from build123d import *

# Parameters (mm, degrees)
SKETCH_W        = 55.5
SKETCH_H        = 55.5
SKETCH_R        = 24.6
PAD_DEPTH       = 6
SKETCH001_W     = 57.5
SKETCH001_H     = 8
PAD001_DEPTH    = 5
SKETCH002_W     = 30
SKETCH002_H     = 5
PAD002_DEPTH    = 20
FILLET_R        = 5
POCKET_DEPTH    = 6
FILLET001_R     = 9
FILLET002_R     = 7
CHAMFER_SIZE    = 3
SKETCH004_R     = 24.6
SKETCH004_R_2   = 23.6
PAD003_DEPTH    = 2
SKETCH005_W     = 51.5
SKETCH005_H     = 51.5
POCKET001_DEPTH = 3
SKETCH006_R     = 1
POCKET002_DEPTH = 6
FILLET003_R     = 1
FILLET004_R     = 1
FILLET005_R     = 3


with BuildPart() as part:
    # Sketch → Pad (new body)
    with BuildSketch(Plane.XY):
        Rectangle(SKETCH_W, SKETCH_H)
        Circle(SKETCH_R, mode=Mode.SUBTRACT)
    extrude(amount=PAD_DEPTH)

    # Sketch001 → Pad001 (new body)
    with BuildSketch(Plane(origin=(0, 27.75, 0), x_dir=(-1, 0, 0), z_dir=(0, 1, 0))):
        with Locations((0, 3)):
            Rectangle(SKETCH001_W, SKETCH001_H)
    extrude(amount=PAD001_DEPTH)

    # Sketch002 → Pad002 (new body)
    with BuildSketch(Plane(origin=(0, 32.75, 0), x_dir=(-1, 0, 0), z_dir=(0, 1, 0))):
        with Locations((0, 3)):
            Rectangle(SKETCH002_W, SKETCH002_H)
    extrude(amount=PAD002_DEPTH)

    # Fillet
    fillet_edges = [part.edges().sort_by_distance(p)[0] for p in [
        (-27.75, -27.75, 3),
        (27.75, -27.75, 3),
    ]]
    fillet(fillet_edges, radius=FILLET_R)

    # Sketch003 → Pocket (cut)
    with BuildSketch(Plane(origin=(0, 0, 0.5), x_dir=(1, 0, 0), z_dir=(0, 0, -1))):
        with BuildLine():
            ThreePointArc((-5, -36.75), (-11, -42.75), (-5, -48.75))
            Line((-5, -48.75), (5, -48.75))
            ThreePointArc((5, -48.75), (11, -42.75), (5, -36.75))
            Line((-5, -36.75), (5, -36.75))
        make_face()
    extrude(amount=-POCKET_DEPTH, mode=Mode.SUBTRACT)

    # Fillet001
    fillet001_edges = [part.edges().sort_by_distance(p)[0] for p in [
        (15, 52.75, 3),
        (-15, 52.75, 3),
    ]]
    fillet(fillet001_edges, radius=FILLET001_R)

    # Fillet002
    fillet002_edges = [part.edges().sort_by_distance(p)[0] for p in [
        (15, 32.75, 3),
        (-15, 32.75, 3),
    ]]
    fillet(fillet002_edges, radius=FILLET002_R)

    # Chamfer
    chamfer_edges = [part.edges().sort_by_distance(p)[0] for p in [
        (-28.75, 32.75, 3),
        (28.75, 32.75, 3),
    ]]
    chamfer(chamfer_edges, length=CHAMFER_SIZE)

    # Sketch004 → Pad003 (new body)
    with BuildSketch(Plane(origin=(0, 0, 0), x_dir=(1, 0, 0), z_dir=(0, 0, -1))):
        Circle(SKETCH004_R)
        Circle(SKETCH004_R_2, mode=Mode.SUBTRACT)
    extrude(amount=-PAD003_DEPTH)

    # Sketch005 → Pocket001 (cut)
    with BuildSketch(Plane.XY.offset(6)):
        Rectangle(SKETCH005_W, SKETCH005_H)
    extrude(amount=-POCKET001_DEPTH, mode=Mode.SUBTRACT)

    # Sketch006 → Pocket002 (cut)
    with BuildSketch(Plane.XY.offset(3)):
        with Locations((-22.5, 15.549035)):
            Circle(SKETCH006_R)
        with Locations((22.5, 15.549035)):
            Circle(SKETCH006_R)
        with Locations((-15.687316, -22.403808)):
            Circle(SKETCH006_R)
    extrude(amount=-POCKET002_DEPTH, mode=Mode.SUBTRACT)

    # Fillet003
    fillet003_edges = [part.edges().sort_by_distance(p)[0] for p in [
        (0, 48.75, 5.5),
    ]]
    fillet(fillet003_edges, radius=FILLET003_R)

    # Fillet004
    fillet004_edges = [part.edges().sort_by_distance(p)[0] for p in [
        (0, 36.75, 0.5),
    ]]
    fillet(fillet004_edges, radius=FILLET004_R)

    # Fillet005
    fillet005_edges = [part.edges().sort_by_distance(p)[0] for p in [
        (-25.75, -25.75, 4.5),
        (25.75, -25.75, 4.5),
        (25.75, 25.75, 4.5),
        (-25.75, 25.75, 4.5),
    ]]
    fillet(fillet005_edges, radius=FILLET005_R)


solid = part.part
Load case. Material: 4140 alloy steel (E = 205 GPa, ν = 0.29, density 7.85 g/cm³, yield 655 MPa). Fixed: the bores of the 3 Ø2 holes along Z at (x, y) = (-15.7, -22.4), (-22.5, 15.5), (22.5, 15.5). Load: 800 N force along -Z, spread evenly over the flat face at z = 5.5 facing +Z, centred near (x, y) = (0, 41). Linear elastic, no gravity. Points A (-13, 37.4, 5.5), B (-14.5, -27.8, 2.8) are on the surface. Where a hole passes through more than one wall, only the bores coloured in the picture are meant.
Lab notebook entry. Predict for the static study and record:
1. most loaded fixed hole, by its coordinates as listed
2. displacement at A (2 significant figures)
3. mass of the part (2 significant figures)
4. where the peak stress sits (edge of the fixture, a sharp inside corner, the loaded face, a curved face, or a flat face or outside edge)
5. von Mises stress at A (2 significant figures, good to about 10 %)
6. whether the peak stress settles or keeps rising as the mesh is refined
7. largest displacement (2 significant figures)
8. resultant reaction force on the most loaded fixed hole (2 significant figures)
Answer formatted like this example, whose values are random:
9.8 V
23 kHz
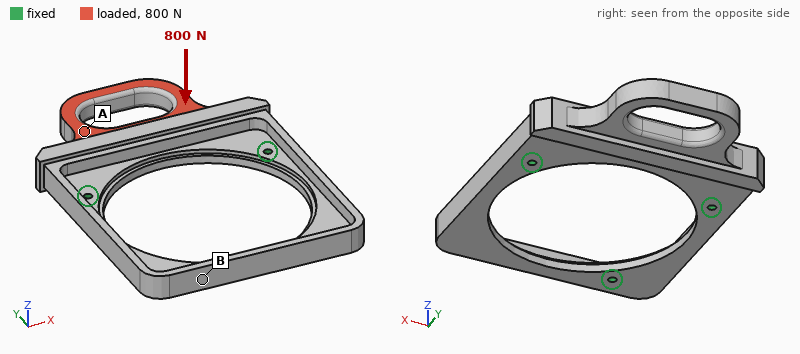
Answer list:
(-22.5, 15.5)
0.19 mm
71 g
edge of the fixture
89 MPa
keeps rising
0.38 mm
550 N
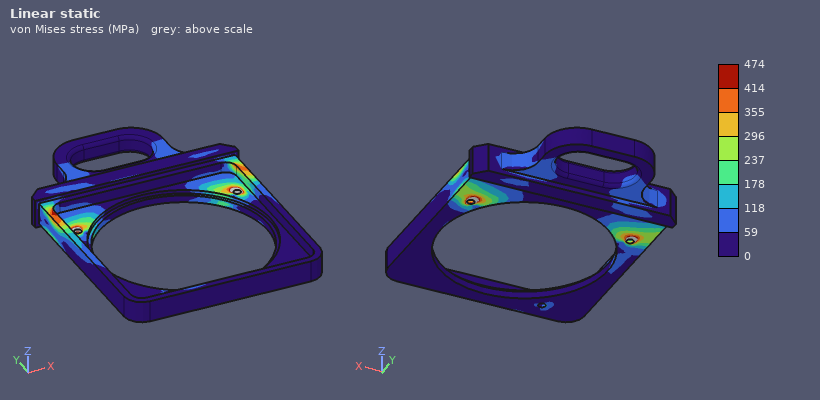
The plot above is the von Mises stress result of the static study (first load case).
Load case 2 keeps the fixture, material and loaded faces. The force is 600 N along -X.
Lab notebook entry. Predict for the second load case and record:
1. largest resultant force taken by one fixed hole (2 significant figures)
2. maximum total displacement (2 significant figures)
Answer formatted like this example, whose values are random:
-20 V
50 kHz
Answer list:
440 N
9.5 µm
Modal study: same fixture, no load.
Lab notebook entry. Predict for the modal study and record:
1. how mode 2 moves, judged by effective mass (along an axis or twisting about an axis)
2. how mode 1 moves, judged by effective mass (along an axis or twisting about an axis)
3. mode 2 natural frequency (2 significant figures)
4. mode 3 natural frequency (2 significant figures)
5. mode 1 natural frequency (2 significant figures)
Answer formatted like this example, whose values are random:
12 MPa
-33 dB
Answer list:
along Z
along Z
2400 Hz
7300 Hz
2000 Hz
